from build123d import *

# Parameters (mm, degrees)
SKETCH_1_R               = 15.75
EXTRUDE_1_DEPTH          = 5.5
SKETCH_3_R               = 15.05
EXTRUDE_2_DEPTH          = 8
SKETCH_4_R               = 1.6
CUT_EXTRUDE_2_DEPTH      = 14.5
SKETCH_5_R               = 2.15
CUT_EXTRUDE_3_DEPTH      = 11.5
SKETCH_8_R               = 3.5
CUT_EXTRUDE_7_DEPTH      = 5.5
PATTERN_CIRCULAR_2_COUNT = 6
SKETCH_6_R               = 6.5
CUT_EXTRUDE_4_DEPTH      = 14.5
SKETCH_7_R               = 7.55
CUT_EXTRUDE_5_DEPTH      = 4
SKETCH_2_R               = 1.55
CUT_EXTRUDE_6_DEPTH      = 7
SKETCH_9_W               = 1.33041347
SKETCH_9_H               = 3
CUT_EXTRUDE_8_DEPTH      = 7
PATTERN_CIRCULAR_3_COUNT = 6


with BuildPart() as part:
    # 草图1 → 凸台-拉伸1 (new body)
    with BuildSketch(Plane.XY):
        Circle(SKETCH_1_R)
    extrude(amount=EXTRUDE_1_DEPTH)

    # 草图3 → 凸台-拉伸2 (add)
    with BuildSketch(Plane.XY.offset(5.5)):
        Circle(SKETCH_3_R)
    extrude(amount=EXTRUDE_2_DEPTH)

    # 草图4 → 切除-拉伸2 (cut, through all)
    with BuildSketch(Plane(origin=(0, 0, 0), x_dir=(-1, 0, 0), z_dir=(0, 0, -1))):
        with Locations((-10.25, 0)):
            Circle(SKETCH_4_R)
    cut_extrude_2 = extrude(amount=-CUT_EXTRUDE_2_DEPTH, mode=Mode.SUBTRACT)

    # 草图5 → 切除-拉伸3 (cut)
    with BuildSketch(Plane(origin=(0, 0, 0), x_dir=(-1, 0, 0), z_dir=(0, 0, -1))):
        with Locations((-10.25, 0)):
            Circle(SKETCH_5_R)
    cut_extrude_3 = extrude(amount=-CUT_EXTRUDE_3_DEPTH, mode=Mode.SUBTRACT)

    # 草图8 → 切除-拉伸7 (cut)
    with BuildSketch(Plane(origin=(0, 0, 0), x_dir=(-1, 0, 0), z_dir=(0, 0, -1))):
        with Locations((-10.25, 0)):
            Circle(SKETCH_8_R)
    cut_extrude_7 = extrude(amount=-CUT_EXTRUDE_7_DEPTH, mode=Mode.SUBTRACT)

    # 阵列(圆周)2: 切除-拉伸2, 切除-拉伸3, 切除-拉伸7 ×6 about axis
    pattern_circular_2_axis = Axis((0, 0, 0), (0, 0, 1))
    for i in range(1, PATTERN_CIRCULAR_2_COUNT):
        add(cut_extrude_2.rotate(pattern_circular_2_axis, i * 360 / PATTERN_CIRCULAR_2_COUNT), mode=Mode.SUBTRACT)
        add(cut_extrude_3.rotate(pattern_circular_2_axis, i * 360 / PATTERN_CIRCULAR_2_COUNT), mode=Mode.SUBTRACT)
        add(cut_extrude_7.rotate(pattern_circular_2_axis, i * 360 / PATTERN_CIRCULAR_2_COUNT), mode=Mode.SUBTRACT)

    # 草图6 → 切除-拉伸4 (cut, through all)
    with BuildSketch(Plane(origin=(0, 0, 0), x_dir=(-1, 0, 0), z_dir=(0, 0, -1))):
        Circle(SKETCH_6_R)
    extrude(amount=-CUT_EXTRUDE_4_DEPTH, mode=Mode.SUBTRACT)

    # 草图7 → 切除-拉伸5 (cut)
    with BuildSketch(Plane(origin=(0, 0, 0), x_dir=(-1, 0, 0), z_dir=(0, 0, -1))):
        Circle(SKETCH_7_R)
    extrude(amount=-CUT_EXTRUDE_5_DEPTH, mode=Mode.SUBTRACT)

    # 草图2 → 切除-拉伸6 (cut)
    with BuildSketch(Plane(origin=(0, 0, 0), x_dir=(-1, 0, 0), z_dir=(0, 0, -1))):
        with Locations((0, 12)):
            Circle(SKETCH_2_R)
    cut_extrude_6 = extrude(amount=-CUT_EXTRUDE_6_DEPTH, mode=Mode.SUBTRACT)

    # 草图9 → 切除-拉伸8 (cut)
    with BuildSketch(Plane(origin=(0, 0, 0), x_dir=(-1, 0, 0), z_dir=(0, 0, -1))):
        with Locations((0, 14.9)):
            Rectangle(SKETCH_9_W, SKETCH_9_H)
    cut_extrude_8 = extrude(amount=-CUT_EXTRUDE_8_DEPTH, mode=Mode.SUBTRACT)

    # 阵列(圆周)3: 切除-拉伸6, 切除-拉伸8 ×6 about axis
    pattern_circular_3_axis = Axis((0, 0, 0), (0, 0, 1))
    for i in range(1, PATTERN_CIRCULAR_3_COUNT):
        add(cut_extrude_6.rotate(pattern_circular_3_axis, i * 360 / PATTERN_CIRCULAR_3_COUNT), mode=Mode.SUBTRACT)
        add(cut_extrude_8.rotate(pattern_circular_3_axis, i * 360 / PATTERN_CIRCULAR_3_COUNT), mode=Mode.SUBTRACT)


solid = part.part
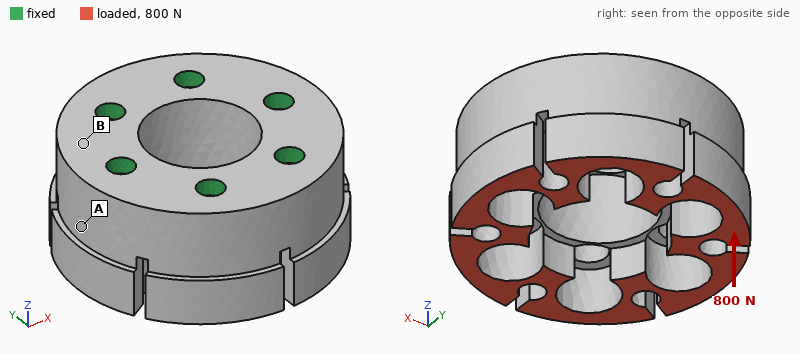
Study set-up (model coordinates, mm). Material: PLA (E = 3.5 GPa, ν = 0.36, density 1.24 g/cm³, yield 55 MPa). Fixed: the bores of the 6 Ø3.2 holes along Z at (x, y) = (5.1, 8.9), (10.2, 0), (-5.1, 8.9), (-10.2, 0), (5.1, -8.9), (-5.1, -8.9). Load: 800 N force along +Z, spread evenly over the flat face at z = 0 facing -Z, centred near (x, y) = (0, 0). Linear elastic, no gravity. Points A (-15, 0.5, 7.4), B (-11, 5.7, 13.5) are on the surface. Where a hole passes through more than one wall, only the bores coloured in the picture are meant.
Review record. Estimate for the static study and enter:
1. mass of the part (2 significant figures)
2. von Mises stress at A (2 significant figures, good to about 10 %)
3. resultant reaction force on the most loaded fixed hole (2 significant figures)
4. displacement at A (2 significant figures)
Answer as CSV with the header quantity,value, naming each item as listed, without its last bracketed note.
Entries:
quantity,value
mass of the part,7.1 g
von Mises stress at A,4.2 MPa
resultant reaction force on the most loaded fixed hole,140 N
displacement at A,18 µm
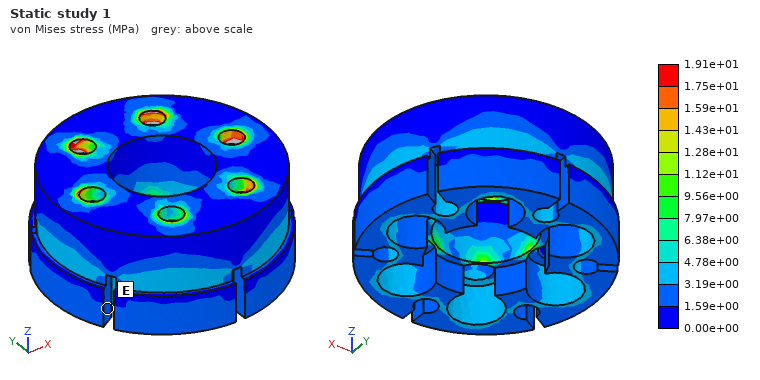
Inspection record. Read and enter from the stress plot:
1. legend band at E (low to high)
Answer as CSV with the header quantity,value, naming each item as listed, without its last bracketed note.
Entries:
quantity,value
legend band at E,1.59e+00 to 3.19e+00 MPa
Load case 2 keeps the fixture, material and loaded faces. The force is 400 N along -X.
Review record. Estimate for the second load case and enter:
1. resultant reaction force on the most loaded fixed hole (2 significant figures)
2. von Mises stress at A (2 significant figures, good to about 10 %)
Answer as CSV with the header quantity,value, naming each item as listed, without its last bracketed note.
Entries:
quantity,value
resultant reaction force on the most loaded fixed hole,140 N
von Mises stress at A,5.3 MPa
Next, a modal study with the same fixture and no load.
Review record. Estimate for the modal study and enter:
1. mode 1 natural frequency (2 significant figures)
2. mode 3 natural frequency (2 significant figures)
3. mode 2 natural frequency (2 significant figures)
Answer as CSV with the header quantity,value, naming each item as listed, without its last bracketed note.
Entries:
quantity,value
mode 1 natural frequency,8800 Hz
mode 3 natural frequency,9700 Hz
mode 2 natural frequency,8800 Hz
